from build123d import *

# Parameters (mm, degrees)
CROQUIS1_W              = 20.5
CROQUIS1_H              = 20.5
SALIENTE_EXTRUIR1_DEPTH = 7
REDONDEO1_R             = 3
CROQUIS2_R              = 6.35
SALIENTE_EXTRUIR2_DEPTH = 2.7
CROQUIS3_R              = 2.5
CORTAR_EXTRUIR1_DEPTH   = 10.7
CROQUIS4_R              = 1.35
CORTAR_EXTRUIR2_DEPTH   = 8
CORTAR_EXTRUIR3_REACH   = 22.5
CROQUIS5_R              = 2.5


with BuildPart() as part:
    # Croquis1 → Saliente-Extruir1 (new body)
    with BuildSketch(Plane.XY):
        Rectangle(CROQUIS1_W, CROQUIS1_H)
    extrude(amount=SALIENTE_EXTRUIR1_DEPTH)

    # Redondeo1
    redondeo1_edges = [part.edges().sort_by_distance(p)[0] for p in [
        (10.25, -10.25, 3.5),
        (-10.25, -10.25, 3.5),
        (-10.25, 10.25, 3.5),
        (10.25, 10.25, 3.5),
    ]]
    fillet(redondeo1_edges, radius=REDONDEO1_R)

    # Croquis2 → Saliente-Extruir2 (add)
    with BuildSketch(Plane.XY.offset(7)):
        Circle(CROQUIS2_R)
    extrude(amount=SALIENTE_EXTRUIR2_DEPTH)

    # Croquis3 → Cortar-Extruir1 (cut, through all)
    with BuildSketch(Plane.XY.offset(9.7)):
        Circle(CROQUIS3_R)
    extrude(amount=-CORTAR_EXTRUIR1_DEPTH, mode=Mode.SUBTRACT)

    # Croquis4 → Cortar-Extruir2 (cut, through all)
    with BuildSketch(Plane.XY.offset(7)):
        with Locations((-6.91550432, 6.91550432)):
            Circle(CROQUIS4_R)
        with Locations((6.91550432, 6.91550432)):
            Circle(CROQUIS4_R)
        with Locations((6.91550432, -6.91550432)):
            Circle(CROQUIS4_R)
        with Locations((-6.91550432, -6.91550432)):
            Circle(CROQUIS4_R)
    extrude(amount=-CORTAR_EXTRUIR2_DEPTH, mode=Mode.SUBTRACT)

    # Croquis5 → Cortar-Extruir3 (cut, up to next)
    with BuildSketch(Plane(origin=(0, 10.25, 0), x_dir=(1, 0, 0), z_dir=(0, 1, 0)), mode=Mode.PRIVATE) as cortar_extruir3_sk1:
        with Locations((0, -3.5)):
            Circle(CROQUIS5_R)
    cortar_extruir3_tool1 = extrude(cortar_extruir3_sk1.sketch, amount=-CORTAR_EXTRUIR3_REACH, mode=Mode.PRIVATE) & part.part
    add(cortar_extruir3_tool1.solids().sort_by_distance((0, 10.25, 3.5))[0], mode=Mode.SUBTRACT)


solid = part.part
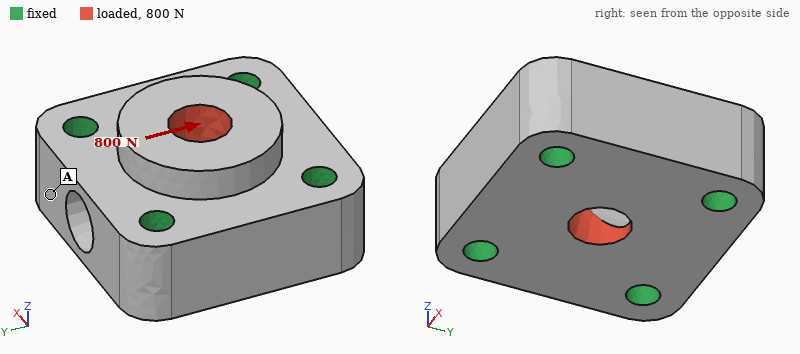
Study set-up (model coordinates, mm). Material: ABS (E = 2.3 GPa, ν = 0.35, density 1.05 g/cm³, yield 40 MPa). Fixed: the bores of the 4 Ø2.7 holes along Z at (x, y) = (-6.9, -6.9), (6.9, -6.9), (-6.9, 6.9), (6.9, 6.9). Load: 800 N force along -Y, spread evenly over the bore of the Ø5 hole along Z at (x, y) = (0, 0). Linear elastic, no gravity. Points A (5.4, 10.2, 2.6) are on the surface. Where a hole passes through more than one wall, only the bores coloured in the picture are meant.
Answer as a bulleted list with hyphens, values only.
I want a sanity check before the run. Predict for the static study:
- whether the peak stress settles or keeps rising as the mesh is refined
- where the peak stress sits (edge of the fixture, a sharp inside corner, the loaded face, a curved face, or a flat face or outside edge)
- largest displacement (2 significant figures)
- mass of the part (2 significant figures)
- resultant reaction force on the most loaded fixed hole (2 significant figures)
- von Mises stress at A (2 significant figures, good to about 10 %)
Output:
- keeps rising
- edge of the fixture
- 39 µm
- 2.9 g
- 240 N
- 2.3 MPa
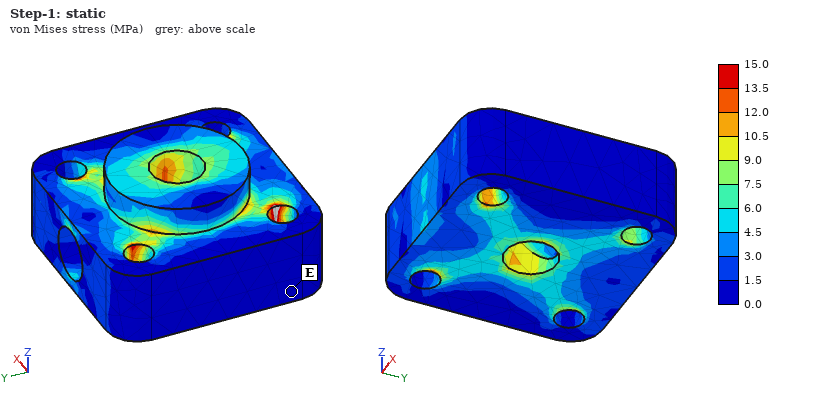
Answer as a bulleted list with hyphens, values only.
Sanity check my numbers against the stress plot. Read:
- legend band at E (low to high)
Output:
- 0.0 to 1.5 MPa
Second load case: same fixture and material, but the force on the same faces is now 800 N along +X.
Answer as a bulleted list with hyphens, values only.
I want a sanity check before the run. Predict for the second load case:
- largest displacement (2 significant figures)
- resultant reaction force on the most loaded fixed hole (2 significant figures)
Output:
- 41 µm
- 260 N
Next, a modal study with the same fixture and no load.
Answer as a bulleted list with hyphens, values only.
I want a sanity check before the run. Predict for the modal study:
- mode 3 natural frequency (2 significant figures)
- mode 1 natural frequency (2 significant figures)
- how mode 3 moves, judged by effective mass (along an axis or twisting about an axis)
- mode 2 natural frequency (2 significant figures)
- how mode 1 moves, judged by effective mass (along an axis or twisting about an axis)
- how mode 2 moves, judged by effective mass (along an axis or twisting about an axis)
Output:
- 28 kHz
- 24 kHz
- along Y
- 27 kHz
- along Z
- along X
